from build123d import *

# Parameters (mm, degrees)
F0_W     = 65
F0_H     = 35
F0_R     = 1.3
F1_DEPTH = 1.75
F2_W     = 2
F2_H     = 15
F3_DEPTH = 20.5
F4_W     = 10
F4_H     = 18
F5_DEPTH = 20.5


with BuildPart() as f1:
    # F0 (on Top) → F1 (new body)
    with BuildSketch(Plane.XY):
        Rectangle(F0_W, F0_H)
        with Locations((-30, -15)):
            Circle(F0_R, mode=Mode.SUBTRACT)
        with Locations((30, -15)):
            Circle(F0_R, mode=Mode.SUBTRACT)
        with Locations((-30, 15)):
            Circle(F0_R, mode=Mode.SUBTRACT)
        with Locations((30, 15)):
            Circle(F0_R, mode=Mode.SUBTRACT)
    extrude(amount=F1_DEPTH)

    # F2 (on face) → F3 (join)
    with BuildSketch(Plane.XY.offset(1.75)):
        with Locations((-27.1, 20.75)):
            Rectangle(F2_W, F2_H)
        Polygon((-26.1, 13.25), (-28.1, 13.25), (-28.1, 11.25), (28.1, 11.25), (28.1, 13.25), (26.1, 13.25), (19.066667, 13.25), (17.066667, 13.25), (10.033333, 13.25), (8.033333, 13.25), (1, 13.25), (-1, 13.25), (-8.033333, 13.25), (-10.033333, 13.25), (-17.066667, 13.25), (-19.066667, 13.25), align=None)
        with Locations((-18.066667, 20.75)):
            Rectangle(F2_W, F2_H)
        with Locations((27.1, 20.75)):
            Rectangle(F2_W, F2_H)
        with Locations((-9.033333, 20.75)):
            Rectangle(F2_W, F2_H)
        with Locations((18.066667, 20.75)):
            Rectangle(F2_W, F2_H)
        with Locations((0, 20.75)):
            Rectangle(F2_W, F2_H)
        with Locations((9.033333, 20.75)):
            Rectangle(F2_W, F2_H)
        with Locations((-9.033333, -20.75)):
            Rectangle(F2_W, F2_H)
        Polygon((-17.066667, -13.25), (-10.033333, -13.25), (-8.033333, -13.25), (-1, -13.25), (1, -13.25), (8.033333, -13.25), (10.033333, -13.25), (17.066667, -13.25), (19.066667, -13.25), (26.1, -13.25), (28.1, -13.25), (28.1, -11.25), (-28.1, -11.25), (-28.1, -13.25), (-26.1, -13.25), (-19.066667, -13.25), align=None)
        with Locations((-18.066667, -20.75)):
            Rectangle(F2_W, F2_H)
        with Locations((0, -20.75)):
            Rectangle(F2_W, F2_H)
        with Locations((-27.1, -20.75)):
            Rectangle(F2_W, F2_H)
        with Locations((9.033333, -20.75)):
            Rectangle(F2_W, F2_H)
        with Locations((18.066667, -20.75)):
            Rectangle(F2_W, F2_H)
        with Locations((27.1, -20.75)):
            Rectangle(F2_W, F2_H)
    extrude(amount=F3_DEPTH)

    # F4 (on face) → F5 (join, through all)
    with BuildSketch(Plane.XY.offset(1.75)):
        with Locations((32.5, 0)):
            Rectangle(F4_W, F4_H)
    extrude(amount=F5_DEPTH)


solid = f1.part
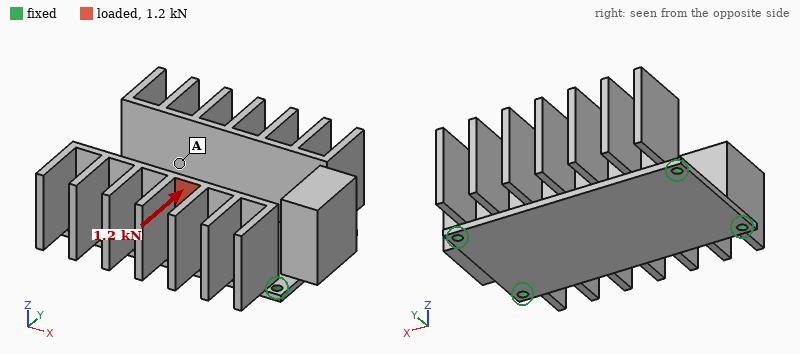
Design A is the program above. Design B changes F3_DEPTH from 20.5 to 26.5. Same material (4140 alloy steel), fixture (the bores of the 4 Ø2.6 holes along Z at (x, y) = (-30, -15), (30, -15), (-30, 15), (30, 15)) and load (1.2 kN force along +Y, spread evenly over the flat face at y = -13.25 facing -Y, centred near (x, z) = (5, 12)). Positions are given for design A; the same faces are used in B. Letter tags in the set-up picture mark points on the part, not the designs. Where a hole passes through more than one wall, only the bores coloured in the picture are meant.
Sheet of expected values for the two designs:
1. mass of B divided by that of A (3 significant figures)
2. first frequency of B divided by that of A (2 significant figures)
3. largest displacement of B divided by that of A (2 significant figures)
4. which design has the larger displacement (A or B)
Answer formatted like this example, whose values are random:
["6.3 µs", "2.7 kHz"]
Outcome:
["1.19", "0.77", "1.3", "B"]
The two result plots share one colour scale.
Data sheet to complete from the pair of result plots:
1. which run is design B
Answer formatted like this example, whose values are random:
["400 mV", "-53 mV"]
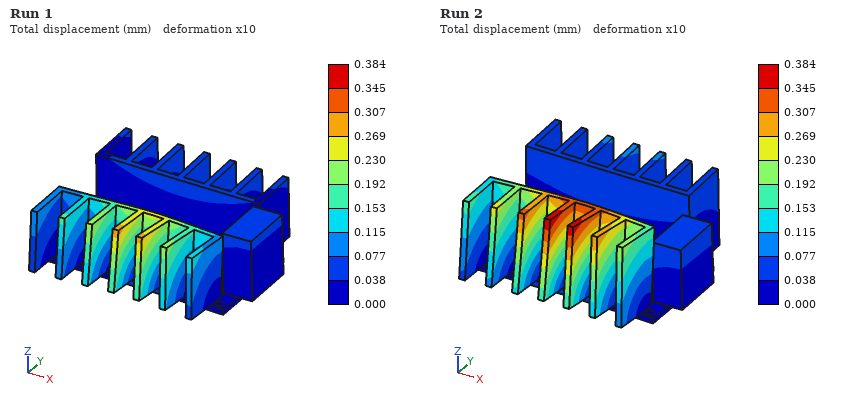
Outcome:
["Run 2"]
